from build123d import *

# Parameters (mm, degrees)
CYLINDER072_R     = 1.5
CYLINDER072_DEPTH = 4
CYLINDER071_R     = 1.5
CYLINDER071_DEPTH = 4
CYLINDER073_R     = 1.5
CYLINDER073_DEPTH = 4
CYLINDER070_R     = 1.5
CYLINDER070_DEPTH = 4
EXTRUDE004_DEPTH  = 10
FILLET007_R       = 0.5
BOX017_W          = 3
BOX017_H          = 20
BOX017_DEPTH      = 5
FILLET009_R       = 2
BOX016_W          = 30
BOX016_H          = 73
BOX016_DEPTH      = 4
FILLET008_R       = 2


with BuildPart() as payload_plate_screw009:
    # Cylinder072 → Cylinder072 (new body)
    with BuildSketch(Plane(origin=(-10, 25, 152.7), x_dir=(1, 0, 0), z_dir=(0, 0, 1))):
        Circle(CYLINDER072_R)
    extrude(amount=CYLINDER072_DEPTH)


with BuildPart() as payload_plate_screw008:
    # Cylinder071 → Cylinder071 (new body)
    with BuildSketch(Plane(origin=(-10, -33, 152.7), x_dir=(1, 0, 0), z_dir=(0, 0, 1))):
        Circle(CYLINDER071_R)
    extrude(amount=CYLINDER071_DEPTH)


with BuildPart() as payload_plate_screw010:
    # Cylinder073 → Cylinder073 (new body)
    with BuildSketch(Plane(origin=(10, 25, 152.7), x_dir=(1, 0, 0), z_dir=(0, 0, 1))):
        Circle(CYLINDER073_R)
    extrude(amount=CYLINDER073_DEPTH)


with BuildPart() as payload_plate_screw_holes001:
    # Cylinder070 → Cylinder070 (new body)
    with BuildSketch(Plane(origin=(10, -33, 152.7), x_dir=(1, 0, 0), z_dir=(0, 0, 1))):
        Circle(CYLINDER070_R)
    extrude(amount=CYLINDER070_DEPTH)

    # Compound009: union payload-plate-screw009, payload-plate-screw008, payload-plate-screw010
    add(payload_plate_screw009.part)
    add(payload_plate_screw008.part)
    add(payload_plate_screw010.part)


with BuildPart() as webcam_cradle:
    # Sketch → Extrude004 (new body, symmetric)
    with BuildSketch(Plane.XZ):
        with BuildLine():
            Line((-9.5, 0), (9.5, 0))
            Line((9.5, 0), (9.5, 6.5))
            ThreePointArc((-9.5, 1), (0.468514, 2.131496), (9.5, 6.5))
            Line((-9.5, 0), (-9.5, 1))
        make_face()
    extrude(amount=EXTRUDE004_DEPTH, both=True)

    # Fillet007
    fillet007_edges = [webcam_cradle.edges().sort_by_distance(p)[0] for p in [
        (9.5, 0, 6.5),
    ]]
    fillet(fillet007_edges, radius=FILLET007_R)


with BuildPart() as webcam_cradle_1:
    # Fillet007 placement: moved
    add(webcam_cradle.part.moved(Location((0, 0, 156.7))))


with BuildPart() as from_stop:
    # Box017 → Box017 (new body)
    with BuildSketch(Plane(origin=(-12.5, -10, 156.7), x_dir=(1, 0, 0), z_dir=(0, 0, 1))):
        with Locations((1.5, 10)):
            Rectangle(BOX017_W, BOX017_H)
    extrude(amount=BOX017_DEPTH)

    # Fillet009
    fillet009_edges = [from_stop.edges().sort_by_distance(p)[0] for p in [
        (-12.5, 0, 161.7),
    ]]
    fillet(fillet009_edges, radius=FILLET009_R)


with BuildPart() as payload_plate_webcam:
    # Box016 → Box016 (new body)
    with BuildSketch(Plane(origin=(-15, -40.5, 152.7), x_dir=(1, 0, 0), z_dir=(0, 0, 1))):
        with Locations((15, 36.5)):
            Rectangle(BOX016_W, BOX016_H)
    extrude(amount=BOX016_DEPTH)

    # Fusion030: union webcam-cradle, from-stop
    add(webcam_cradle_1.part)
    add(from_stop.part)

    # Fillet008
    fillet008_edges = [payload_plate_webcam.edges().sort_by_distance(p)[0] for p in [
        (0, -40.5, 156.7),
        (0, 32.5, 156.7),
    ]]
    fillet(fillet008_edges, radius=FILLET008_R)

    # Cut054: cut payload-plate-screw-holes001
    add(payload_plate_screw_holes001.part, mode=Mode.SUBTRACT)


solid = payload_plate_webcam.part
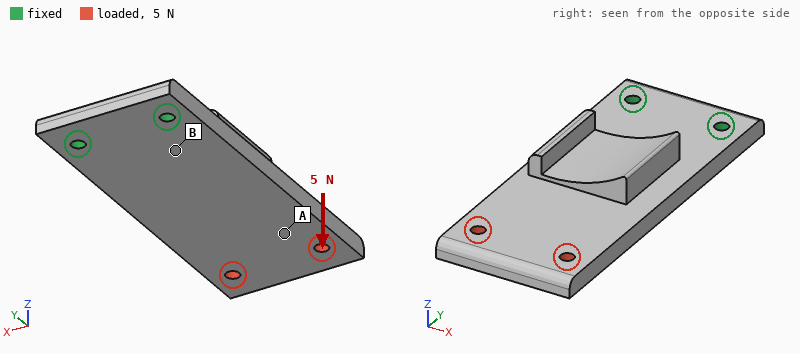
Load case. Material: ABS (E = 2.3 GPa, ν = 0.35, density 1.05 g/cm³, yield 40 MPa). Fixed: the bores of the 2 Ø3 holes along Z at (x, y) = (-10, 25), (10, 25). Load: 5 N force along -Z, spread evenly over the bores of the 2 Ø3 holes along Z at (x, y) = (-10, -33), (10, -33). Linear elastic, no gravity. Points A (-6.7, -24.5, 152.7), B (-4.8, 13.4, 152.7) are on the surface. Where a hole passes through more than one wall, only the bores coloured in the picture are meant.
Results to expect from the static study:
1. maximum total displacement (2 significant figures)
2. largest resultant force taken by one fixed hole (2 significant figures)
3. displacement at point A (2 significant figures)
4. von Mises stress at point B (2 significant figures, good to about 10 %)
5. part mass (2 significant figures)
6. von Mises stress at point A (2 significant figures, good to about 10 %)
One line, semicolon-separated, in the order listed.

0.83 mm; 2.6 N; 0.56 mm; 2.6 MPa; 10 g; 0.52 MPa
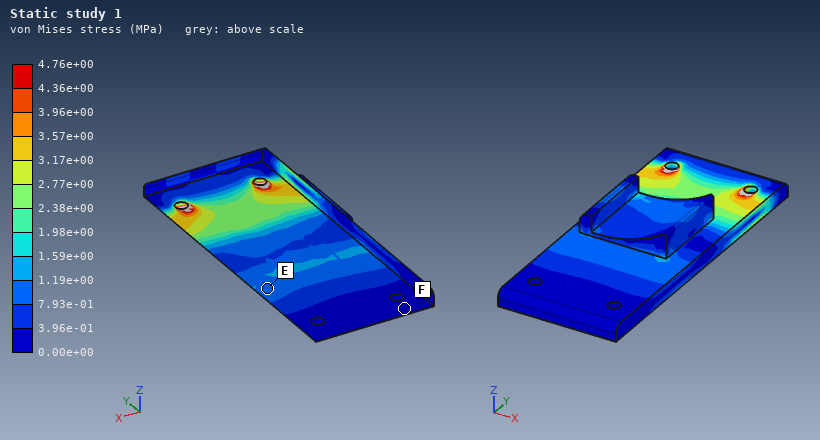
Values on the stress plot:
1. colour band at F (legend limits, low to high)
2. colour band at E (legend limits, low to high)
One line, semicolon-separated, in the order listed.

0.00e+00 to 3.96e-01 MPa; 7.93e-01 to 1.19e+00 MPa
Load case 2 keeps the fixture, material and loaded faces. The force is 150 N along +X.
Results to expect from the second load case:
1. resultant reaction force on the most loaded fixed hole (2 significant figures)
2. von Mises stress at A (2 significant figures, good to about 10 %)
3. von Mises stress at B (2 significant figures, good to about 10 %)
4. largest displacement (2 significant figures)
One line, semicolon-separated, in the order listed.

420 N; 2.9 MPa; 5.4 MPa; 0.71 mm
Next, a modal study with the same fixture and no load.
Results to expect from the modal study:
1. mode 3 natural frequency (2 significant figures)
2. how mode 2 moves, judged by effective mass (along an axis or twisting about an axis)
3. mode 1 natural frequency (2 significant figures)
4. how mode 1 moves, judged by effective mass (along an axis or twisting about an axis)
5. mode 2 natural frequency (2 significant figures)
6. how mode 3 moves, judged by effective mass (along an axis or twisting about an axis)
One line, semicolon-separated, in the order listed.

1400 Hz; twisting about Y; 240 Hz; along Z; 1200 Hz; along X
